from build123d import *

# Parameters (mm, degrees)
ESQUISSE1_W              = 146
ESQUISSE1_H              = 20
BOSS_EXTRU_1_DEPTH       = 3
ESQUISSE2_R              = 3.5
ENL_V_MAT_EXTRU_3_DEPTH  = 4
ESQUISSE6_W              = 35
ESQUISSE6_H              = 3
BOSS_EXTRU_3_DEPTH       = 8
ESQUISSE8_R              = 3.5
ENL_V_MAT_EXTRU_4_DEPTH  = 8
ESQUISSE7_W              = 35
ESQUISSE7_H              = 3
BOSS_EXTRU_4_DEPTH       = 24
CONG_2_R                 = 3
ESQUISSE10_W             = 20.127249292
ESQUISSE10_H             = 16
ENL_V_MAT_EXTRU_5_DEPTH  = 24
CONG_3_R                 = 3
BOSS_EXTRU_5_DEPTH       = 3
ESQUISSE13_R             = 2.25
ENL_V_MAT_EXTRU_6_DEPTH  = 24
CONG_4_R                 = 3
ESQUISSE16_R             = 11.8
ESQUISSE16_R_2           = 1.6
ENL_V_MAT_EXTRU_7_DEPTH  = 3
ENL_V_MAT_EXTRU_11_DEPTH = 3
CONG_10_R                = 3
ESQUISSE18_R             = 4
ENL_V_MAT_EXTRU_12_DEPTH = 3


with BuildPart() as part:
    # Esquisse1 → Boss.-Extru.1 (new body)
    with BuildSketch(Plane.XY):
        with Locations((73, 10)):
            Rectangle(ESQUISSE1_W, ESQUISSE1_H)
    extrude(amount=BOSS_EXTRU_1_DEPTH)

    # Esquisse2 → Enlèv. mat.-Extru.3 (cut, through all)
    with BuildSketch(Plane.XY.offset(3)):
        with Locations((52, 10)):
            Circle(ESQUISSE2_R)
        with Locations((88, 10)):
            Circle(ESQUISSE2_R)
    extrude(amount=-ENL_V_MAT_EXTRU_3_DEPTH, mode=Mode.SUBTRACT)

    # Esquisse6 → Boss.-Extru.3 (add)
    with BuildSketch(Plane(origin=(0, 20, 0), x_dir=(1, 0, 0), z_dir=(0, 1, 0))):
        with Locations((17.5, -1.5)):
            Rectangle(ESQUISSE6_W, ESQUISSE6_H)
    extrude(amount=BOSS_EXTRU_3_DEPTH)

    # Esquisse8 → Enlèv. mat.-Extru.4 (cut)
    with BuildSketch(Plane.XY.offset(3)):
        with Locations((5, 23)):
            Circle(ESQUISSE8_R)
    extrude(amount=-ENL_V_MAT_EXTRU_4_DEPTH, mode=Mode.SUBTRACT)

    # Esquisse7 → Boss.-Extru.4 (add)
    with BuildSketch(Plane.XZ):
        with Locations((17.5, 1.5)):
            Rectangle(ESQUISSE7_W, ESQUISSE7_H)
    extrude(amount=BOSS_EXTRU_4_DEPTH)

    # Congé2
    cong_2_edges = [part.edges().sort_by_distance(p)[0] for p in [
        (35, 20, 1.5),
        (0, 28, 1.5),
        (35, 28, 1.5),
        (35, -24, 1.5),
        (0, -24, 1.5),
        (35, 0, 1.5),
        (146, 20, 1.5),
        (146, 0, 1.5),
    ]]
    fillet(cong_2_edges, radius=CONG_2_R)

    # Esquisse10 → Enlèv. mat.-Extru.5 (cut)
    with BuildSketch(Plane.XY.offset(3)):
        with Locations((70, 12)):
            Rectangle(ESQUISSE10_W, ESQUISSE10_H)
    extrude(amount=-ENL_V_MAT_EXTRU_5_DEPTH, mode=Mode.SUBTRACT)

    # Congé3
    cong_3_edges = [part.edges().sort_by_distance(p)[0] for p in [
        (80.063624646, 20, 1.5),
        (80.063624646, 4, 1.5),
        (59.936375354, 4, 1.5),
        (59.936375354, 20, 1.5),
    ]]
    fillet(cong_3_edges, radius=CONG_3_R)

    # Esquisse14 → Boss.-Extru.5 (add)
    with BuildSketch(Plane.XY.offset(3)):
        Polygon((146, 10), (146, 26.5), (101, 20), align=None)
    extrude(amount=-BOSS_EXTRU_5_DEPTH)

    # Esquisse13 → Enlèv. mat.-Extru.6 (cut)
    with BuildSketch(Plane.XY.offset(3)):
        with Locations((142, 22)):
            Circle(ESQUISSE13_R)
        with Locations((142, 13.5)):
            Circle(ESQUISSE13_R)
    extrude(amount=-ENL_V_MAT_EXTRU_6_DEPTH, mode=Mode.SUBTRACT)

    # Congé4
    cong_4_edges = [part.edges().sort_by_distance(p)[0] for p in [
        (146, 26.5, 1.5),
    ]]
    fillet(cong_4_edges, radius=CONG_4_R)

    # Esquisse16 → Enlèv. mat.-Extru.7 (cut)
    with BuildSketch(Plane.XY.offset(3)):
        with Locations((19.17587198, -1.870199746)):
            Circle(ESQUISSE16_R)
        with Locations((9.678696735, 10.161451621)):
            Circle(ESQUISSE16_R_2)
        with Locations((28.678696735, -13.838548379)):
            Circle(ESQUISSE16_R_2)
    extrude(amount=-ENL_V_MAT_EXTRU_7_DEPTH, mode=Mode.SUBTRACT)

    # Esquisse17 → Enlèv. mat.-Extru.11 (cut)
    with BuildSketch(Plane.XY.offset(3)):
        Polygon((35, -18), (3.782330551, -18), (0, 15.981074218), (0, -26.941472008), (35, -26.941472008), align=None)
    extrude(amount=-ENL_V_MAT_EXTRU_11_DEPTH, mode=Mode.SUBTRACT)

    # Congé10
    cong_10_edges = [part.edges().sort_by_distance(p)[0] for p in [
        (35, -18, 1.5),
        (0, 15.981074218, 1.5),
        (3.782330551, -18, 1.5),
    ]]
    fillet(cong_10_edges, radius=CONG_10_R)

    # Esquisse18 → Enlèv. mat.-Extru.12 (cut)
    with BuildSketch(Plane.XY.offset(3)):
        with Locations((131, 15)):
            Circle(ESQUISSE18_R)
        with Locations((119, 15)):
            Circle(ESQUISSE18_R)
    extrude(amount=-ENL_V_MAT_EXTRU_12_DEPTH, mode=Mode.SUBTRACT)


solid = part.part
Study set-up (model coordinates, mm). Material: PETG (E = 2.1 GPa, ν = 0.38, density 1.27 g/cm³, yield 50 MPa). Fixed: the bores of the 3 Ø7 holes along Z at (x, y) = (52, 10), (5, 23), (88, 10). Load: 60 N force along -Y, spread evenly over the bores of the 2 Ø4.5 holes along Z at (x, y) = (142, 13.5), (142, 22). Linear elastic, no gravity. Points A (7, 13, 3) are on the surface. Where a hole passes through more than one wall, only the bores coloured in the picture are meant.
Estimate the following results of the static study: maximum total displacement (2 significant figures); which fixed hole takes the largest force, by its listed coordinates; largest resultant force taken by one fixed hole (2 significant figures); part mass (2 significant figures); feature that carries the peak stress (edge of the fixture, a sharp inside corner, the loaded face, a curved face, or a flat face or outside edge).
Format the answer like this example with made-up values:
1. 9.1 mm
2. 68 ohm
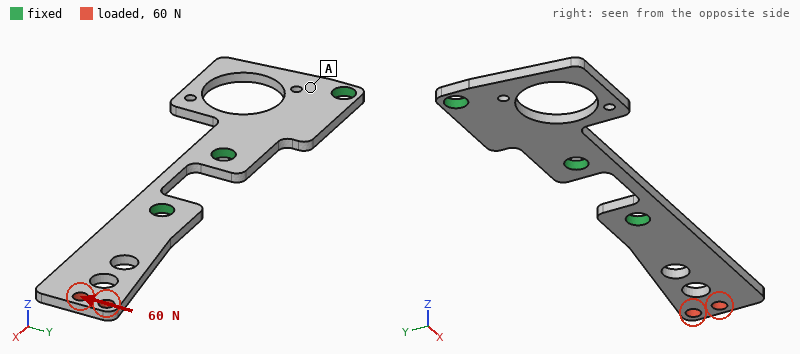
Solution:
1. 1.3 mm
2. (88, 10)
3. 72 N
4. 11 g
5. edge of the fixture
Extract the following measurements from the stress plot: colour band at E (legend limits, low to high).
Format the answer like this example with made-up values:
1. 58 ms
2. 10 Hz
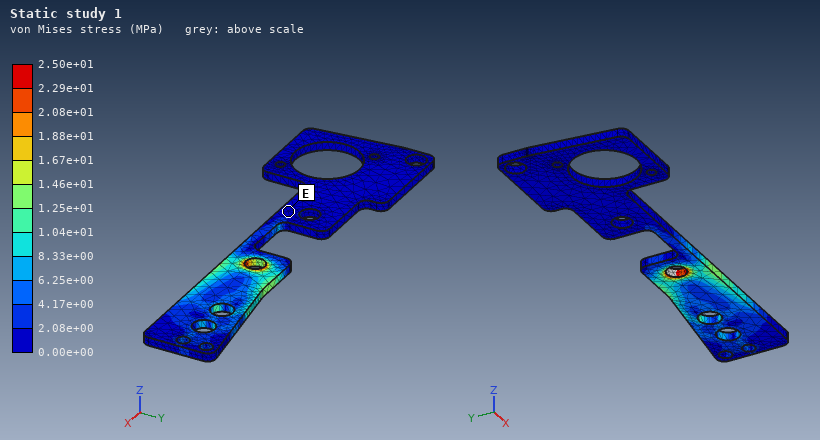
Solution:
1. 0.00e+00 to 2.08e+00 MPa
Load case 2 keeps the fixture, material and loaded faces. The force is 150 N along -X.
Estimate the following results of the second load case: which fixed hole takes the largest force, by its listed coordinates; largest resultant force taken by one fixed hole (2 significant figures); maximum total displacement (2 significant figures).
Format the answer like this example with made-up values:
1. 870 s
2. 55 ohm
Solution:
1. (88, 10)
2. 160 N
3. 0.62 mm
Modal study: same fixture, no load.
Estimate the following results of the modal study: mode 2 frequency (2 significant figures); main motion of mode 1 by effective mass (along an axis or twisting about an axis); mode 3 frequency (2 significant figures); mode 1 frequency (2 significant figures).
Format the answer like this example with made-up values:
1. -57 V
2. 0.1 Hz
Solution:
1. 490 Hz
2. along Z
3. 790 Hz
4. 200 Hz
